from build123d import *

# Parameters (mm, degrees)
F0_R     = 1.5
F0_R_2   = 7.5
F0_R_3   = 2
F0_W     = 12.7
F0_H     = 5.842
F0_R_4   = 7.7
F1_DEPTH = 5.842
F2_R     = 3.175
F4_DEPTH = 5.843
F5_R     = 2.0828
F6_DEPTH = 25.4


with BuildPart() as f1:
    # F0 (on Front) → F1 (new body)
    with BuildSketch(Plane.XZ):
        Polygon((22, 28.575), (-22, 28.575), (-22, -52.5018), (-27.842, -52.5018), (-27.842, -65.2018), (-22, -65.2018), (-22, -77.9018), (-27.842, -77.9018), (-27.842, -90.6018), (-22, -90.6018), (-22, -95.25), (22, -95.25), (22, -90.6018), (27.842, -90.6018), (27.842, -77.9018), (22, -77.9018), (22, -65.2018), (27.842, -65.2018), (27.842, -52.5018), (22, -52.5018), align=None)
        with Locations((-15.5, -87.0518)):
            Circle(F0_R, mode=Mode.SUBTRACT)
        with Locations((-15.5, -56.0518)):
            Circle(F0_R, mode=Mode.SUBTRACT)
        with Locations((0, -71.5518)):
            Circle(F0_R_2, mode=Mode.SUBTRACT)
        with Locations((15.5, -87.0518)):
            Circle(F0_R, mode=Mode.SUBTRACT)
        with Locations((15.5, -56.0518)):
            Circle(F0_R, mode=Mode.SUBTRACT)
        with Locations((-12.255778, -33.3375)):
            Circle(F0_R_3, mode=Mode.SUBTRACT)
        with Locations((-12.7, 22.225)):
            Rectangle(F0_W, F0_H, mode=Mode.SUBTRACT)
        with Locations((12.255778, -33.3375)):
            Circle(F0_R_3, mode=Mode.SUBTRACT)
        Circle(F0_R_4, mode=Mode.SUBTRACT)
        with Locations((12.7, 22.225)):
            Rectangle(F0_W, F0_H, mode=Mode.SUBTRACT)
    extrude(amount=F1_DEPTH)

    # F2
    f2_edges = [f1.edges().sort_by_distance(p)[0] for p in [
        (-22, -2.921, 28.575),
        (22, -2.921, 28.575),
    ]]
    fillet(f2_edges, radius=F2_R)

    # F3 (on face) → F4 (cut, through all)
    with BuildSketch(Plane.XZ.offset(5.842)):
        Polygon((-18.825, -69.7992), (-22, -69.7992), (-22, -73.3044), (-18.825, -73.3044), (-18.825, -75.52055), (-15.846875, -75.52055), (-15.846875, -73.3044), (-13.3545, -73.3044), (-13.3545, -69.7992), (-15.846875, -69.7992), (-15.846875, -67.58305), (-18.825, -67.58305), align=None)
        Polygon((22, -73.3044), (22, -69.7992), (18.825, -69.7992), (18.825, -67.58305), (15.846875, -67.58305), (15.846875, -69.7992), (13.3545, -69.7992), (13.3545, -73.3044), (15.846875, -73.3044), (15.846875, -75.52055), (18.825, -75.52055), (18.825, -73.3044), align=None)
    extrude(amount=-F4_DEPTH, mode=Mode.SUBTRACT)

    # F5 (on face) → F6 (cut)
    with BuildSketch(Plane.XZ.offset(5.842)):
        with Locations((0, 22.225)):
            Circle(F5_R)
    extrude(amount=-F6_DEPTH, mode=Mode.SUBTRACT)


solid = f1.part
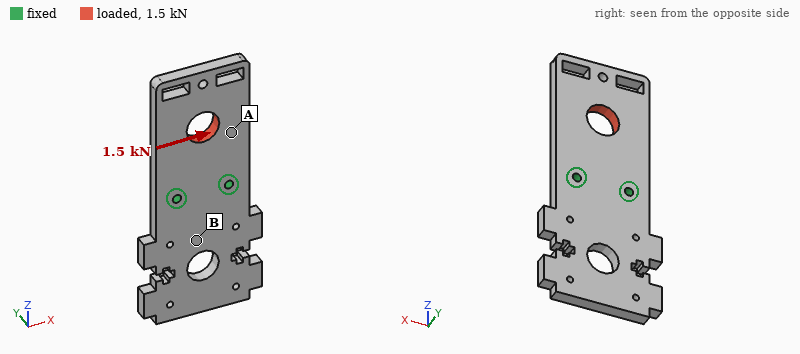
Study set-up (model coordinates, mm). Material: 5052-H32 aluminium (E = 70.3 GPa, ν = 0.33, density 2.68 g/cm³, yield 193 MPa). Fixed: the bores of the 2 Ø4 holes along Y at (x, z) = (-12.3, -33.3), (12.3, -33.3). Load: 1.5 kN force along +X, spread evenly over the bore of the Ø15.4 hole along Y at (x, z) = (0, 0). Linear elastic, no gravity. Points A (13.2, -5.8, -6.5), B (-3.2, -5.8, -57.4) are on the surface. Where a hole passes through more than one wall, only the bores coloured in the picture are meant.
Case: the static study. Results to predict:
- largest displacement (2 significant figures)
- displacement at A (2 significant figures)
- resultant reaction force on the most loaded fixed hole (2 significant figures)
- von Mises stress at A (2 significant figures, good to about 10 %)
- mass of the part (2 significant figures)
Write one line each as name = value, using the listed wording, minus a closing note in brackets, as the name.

largest displacement = 35 µm
displacement at A = 16 µm
resultant reaction force on the most loaded fixed hole = 2.0 kN
von Mises stress at A = 12 MPa
mass of the part = 79 g
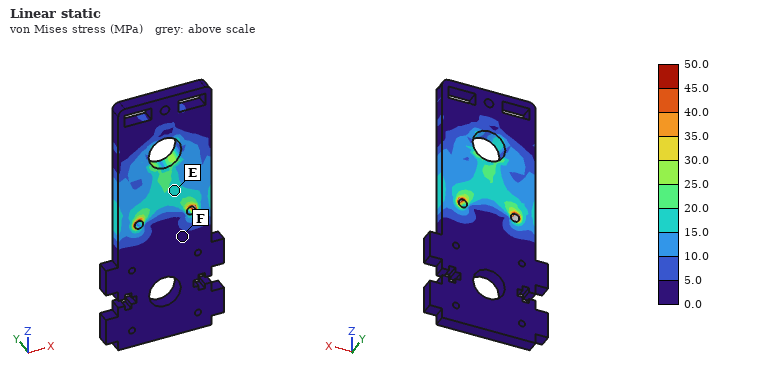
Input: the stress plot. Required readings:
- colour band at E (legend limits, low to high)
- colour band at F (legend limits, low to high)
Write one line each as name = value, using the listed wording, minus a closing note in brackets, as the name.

colour band at E = 15.0 to 20.0 MPa
colour band at F = 0.0 to 5.0 MPa
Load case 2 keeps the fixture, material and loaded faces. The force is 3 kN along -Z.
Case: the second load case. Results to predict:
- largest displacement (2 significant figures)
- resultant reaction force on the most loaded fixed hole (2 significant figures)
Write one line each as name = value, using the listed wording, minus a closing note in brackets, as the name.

largest displacement = 11 µm
resultant reaction force on the most loaded fixed hole = 1.5 kN
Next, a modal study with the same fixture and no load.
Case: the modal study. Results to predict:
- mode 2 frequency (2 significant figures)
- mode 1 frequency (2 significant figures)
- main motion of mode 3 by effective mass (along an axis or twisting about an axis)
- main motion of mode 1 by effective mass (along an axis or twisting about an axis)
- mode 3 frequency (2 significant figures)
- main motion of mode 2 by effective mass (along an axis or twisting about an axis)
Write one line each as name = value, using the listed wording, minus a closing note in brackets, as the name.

mode 2 frequency = 1400 Hz
mode 1 frequency = 1100 Hz
main motion of mode 3 by effective mass = twisting about Z
main motion of mode 1 by effective mass = along Y
mode 3 frequency = 2600 Hz
main motion of mode 2 by effective mass = along Y
